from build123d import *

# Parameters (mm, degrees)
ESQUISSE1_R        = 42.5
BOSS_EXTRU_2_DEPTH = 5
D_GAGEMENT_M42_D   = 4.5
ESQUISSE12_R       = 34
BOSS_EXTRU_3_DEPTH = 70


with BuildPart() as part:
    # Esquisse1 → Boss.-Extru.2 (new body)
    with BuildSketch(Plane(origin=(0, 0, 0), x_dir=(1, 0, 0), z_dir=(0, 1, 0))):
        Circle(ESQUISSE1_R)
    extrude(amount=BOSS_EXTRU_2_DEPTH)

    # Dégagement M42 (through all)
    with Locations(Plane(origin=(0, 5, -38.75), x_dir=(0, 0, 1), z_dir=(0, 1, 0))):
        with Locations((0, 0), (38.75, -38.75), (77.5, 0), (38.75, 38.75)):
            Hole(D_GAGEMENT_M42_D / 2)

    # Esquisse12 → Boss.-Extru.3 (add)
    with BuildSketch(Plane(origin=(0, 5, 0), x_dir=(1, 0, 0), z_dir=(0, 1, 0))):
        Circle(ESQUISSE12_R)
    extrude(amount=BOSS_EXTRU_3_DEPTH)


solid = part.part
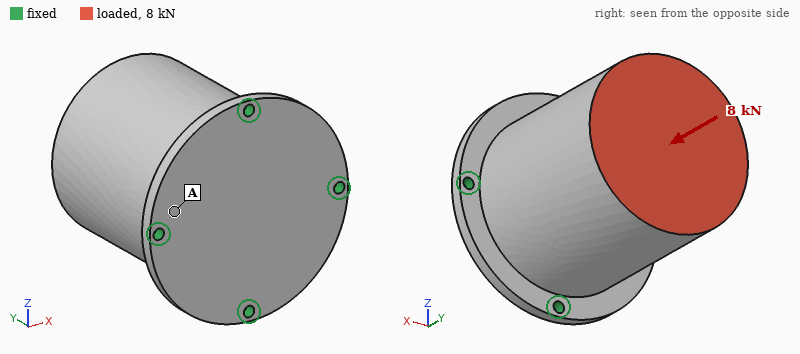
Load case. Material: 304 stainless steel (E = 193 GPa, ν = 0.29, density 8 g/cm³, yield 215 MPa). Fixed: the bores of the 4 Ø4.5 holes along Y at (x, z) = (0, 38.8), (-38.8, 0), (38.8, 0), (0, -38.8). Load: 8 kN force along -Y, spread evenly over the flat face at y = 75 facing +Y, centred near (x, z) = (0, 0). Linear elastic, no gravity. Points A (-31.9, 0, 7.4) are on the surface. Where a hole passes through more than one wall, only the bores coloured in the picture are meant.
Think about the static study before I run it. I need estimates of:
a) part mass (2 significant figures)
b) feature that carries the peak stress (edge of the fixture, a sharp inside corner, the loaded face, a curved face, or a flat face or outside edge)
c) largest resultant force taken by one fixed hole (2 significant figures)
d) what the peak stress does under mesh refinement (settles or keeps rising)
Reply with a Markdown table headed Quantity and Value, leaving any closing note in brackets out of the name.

| Quantity | Value |
|---|---|
| part mass | 2.3 kg |
| feature that carries the peak stress | edge of the fixture |
| largest resultant force taken by one fixed hole | 2.2 kN |
| what the peak stress does under mesh refinement | keeps rising |
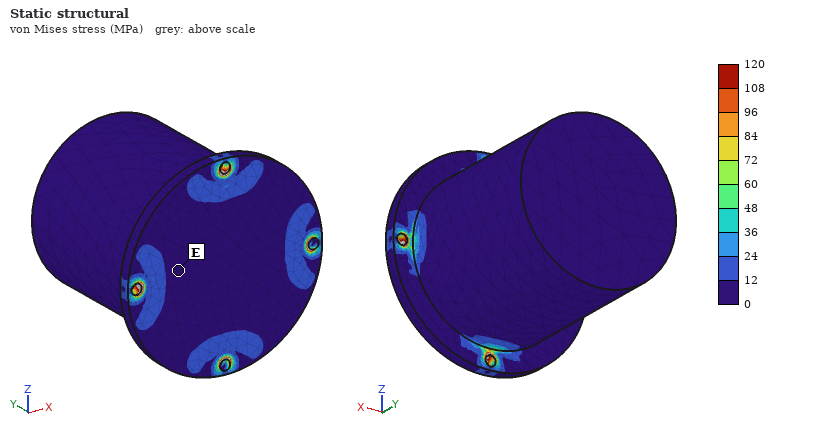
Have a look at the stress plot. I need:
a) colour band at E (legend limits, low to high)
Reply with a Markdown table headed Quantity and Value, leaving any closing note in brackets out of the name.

| Quantity | Value |
|---|---|
| colour band at E | 0 to 12 MPa |
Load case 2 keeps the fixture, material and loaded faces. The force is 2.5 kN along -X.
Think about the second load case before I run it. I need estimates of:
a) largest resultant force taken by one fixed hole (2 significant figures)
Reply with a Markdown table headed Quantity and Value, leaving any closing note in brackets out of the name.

| Quantity | Value |
|---|---|
| largest resultant force taken by one fixed hole | 2.7 kN |
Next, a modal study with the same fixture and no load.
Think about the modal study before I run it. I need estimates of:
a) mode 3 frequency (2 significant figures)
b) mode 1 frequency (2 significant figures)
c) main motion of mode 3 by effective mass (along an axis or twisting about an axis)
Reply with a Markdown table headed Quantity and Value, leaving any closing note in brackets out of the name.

| Quantity | Value |
|---|---|
| mode 3 frequency | 4200 Hz |
| mode 1 frequency | 2400 Hz |
| main motion of mode 3 by effective mass | along Y |
